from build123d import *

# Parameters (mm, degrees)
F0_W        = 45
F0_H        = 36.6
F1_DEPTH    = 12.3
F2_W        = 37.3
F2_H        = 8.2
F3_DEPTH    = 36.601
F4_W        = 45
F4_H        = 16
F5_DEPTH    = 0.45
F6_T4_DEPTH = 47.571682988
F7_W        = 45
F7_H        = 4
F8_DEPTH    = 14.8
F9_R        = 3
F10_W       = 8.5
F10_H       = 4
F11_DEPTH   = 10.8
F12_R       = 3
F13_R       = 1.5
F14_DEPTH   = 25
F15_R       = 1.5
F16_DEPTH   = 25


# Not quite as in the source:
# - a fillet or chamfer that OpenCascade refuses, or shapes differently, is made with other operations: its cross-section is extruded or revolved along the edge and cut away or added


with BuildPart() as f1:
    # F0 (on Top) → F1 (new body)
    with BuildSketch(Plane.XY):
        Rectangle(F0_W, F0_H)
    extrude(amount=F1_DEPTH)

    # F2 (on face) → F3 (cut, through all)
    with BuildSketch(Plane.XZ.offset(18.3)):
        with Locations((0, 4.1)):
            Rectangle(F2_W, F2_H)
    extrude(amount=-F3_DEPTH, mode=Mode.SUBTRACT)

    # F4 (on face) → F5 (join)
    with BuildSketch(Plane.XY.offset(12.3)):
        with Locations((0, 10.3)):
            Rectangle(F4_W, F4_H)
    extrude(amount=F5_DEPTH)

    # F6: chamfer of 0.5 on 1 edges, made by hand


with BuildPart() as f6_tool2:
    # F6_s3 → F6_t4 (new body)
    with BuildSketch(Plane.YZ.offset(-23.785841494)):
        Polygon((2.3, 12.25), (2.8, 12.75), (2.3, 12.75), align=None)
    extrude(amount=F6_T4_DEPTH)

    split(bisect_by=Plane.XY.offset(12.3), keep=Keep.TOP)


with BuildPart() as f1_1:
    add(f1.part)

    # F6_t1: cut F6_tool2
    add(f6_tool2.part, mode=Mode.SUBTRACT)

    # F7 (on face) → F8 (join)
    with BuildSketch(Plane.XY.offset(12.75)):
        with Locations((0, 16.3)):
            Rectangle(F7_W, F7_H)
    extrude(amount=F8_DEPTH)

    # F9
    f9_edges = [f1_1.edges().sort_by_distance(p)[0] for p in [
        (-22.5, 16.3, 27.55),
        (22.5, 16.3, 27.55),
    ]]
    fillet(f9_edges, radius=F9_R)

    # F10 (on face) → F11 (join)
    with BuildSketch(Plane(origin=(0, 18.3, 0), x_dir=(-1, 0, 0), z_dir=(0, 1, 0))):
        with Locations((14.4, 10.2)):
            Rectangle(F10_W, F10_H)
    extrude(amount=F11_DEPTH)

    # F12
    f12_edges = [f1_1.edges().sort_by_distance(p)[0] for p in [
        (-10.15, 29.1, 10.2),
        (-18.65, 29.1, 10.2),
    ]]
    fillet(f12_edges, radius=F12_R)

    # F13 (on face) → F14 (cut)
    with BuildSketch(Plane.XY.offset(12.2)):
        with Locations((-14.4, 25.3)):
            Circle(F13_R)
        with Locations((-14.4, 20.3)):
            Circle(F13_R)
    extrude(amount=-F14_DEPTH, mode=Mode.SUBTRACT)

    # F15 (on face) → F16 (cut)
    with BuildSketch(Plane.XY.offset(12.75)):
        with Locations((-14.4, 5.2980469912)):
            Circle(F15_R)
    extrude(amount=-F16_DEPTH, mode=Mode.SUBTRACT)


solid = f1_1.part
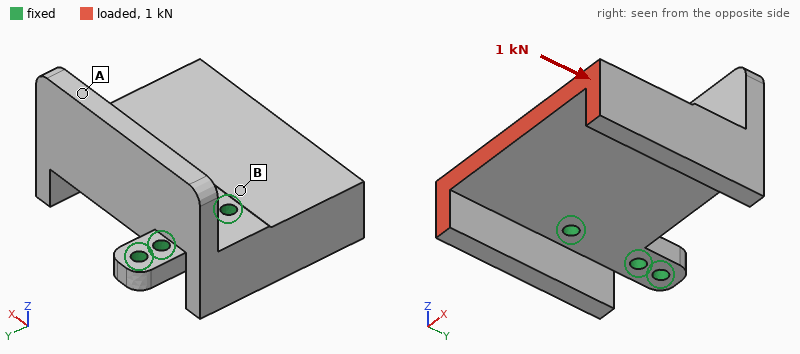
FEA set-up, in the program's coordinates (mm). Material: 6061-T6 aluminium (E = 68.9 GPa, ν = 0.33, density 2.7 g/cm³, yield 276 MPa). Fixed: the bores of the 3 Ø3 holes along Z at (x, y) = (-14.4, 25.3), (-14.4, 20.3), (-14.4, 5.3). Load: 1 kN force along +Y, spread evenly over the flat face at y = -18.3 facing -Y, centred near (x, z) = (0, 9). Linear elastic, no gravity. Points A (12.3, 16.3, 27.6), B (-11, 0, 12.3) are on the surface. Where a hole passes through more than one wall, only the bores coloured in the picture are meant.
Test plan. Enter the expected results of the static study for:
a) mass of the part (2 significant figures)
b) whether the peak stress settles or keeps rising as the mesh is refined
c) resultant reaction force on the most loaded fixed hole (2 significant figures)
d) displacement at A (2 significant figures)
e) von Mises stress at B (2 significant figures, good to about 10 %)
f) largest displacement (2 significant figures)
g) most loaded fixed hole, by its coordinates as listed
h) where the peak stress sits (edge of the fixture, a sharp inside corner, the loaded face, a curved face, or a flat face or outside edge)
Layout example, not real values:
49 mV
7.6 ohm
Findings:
33 g
keeps rising
1.1 kN
11 µm
17 MPa
55 µm
(-14.4, 5.3)
edge of the fixture
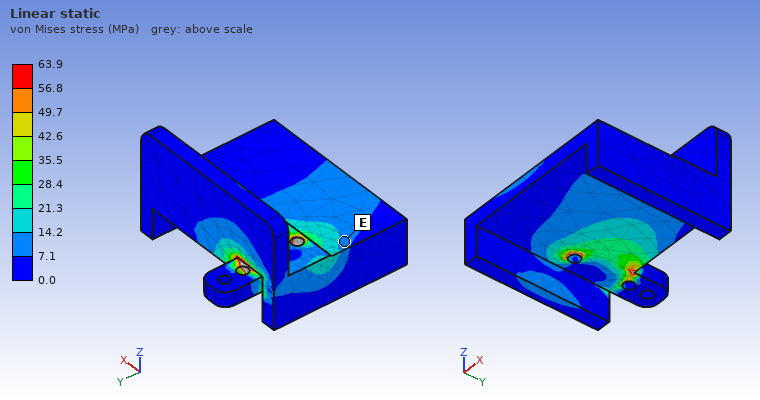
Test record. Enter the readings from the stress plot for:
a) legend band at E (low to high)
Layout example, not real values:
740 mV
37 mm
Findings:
7.1 to 14.2 MPa
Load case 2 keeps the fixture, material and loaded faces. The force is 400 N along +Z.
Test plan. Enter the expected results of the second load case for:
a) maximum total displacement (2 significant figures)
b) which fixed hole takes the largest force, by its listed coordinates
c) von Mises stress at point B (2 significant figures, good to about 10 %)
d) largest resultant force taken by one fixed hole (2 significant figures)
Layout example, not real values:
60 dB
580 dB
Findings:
0.25 mm
(-14.4, 5.3)
61 MPa
860 N
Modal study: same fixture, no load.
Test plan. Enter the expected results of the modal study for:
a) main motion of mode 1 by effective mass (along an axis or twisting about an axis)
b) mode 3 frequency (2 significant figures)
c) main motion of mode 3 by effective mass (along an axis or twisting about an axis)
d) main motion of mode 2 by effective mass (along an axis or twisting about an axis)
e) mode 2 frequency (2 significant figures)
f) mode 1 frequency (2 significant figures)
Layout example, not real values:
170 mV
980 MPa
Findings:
along Z
5200 Hz
along Y
twisting about X
4000 Hz
2200 Hz
